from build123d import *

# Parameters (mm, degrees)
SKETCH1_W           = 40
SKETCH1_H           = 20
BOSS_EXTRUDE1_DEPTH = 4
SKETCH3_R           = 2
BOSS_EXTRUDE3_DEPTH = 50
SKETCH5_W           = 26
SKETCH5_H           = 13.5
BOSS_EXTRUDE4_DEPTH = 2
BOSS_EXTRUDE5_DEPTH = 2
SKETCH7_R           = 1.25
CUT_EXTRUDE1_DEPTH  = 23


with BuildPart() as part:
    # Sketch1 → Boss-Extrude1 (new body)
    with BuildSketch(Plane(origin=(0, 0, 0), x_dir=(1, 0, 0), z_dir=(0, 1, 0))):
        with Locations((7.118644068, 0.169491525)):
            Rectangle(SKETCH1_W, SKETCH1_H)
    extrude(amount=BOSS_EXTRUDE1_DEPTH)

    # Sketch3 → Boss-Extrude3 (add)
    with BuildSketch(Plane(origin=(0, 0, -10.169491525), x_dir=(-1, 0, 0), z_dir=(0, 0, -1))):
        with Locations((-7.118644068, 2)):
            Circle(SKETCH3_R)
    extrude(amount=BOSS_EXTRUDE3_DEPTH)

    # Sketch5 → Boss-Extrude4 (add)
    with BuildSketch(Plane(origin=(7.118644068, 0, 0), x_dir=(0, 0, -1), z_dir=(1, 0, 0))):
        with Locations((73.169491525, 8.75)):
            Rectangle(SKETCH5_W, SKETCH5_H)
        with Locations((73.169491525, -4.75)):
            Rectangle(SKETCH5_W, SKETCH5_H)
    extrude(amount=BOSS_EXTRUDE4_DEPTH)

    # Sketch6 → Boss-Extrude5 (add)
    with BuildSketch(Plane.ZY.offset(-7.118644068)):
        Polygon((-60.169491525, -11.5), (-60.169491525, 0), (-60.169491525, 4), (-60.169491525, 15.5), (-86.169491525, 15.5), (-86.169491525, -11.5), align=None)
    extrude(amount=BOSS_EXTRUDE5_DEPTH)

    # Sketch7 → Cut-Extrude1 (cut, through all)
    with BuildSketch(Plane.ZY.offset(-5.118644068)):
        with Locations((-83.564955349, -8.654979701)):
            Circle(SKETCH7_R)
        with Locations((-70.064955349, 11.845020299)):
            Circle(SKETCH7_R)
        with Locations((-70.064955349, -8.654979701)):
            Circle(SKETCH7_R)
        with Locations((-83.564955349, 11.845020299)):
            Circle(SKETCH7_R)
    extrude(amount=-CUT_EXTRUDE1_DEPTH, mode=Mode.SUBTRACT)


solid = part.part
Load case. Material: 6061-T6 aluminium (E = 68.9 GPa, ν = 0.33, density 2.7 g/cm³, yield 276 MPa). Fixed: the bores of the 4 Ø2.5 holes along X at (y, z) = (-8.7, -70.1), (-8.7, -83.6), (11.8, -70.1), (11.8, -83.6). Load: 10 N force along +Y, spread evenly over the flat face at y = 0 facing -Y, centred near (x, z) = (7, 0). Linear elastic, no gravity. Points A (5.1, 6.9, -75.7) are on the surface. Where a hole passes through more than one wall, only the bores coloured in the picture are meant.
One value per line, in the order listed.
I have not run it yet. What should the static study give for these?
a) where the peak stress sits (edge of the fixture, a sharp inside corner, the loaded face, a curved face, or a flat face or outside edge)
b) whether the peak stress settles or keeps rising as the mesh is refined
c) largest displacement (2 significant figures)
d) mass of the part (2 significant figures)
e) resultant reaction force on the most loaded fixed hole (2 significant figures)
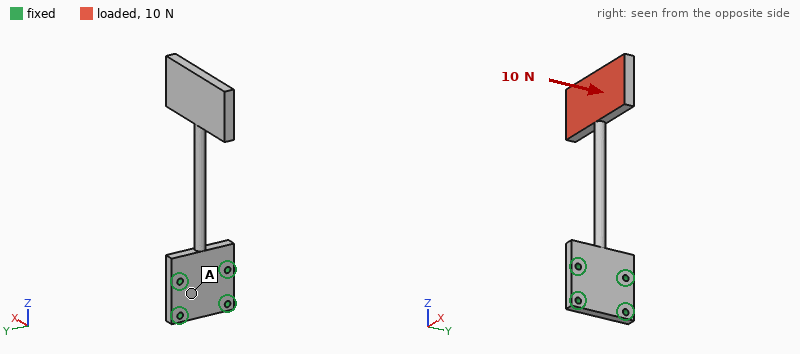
a sharp inside corner
keeps rising
1.1 mm
18 g
31 N
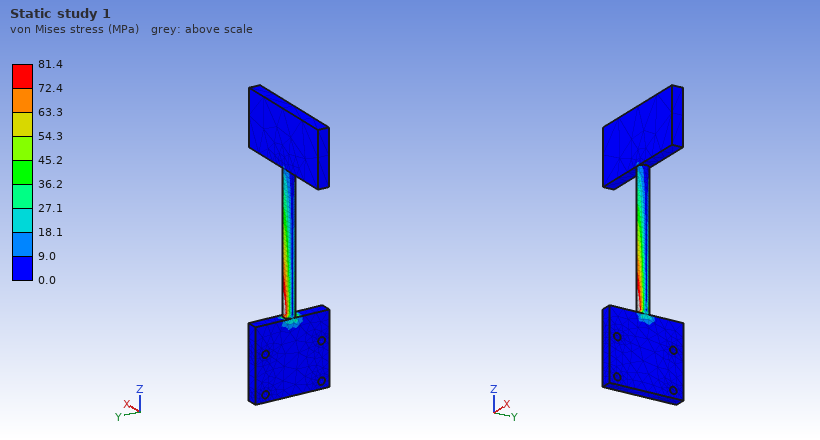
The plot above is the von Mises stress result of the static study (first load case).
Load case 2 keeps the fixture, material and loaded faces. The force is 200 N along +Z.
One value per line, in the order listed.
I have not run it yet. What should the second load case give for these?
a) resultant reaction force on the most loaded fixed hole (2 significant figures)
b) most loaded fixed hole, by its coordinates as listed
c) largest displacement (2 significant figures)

90 N
(-8.7, -70.1)
1.1 mm
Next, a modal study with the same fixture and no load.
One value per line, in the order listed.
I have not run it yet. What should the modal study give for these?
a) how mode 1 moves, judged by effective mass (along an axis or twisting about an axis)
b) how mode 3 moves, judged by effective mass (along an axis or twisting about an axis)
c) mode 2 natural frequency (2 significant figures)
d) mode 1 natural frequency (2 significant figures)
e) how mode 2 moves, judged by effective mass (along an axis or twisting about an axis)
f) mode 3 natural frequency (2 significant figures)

along X
twisting about Z
180 Hz
170 Hz
along Y
520 Hz
